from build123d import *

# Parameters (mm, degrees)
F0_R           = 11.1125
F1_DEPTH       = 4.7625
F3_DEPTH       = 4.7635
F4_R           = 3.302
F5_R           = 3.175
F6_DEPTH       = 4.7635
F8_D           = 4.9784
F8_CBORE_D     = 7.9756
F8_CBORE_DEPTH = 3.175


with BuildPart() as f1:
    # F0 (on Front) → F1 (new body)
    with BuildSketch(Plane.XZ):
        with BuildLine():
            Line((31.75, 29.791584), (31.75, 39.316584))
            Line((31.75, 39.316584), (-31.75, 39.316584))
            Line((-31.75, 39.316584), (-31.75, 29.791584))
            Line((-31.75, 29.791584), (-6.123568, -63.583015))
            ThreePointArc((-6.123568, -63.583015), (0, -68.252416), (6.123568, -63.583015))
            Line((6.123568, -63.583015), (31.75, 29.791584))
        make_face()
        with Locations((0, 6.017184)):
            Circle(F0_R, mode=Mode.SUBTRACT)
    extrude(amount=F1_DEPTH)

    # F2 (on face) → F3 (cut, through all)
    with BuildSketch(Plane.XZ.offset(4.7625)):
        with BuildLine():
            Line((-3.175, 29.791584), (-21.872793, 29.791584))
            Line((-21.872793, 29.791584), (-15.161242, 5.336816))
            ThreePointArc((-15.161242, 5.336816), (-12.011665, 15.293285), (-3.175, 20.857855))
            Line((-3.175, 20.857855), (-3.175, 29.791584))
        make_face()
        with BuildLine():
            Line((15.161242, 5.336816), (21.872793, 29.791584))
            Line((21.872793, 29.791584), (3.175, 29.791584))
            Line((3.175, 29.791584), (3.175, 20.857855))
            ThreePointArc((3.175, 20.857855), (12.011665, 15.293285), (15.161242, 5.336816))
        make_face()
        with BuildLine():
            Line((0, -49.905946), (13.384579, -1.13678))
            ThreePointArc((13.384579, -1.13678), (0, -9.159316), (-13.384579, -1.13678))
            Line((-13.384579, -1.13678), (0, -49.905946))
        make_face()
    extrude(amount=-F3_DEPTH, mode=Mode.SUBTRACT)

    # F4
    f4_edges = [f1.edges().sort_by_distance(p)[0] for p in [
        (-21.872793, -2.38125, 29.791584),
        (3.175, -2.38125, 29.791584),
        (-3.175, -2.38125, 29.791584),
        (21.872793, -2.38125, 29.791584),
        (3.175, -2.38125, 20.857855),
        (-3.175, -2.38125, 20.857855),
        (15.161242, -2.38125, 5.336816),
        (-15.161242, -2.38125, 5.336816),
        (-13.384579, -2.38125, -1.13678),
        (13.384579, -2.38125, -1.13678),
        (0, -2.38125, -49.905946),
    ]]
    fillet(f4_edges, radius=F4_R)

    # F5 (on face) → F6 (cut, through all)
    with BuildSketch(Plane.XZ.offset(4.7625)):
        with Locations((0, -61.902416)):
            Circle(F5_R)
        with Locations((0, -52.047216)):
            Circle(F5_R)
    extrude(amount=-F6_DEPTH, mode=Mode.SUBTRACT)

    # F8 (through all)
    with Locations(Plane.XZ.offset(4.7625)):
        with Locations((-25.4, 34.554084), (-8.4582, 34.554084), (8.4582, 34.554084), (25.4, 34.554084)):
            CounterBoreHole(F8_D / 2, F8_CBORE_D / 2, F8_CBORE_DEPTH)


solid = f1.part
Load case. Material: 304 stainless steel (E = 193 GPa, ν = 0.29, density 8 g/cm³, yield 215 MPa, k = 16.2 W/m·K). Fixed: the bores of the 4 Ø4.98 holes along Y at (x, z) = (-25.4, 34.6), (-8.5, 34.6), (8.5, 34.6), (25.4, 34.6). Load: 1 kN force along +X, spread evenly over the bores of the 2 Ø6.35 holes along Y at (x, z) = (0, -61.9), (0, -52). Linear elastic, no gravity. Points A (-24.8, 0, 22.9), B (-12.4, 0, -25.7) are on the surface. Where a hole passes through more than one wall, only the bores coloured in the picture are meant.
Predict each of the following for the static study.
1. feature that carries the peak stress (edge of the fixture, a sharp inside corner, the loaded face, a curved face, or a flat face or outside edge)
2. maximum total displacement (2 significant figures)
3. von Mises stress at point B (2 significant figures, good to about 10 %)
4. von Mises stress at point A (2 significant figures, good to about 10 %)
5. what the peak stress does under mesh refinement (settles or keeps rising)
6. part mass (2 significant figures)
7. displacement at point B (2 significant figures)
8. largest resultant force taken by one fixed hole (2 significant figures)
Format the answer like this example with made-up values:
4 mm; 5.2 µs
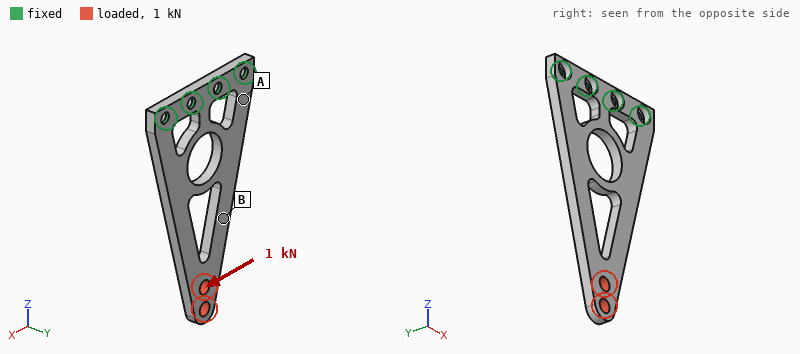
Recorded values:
edge of the fixture; 73 µm; 34 MPa; 54 MPa; keeps rising; 100 g; 38 µm; 1.7 kN
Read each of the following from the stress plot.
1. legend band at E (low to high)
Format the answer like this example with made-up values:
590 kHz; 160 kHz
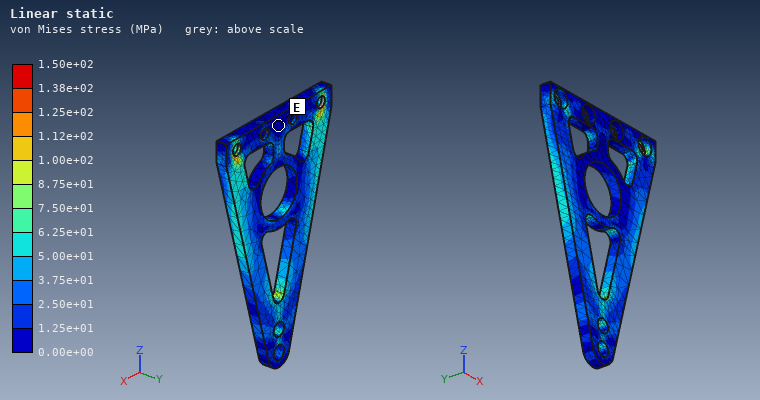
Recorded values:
0.00e+00 to 1.25e+01 MPa
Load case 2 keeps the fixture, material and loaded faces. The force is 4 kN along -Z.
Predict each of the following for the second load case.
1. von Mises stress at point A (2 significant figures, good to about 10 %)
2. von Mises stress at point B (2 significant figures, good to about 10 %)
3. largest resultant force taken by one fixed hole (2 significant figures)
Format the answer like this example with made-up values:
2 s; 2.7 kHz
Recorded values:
40 MPa; 45 MPa; 1.7 kN
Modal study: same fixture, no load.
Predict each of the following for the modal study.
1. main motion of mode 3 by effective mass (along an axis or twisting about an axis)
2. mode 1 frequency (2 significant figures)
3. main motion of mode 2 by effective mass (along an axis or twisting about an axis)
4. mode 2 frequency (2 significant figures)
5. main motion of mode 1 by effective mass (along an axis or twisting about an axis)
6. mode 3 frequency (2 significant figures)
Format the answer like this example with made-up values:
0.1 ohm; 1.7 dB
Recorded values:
twisting about Z; 420 Hz; along Y; 2200 Hz; along Y; 2400 Hz
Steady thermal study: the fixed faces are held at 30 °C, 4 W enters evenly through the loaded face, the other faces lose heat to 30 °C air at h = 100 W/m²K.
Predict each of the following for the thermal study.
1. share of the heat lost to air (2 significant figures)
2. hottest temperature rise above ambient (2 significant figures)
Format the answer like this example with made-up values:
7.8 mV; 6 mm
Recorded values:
100 %; 39 K
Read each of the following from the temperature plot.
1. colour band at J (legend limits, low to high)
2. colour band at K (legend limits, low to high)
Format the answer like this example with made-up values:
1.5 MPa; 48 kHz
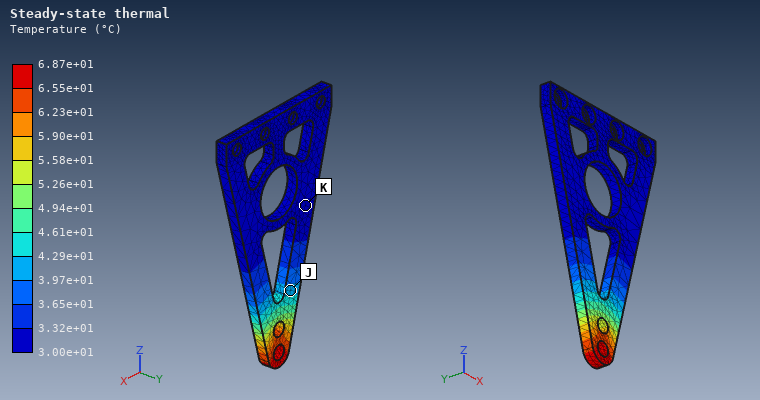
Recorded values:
3.97e+01 to 4.29e+01 °C; 3.00e+01 to 3.32e+01 °C
